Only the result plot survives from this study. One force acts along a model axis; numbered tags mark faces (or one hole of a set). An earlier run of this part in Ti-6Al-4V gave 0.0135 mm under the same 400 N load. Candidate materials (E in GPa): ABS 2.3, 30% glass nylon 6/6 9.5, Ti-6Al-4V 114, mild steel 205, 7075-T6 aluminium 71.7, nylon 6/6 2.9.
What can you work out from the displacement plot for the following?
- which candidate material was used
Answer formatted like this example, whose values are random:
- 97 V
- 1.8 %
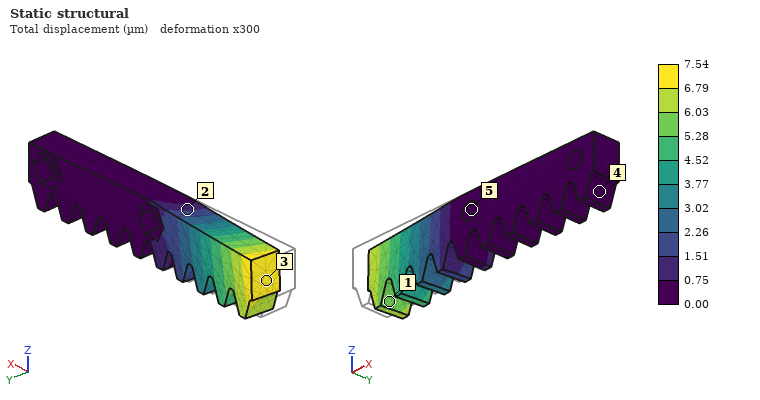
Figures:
- mild steel
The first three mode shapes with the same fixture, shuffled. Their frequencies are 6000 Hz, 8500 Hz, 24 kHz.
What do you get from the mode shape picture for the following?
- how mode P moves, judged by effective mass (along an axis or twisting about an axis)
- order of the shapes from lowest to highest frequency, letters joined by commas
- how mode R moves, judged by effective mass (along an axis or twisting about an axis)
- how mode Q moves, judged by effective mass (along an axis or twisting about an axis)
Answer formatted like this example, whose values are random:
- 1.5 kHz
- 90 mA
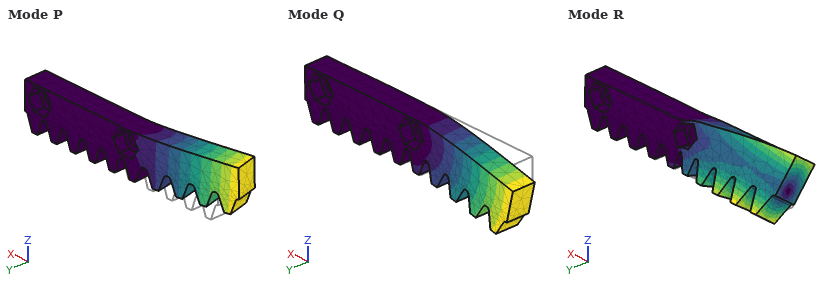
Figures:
- along Y
- P, Q, R
- twisting about X
- along Z
